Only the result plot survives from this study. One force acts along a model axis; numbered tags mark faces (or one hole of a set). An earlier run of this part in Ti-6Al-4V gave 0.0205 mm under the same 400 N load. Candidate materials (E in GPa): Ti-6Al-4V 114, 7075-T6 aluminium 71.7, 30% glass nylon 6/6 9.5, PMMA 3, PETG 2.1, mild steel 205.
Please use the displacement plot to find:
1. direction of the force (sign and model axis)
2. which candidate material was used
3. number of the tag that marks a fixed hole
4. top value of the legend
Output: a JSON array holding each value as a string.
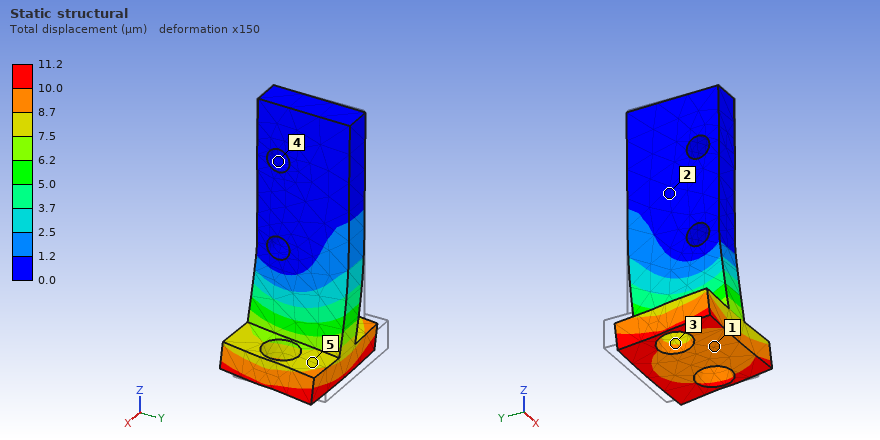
["-Y", "mild steel", "4", "11.2 µm"]
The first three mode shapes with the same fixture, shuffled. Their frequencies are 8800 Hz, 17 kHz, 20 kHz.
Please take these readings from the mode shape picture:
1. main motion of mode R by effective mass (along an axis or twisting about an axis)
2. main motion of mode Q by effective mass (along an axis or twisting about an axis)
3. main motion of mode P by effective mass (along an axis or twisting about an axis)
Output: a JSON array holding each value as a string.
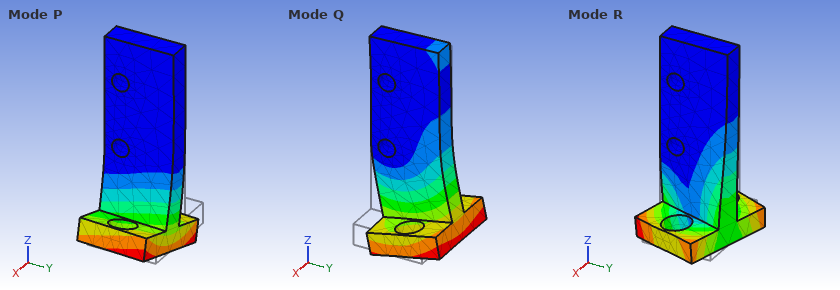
["twisting about Z", "along Y", "along X"]
